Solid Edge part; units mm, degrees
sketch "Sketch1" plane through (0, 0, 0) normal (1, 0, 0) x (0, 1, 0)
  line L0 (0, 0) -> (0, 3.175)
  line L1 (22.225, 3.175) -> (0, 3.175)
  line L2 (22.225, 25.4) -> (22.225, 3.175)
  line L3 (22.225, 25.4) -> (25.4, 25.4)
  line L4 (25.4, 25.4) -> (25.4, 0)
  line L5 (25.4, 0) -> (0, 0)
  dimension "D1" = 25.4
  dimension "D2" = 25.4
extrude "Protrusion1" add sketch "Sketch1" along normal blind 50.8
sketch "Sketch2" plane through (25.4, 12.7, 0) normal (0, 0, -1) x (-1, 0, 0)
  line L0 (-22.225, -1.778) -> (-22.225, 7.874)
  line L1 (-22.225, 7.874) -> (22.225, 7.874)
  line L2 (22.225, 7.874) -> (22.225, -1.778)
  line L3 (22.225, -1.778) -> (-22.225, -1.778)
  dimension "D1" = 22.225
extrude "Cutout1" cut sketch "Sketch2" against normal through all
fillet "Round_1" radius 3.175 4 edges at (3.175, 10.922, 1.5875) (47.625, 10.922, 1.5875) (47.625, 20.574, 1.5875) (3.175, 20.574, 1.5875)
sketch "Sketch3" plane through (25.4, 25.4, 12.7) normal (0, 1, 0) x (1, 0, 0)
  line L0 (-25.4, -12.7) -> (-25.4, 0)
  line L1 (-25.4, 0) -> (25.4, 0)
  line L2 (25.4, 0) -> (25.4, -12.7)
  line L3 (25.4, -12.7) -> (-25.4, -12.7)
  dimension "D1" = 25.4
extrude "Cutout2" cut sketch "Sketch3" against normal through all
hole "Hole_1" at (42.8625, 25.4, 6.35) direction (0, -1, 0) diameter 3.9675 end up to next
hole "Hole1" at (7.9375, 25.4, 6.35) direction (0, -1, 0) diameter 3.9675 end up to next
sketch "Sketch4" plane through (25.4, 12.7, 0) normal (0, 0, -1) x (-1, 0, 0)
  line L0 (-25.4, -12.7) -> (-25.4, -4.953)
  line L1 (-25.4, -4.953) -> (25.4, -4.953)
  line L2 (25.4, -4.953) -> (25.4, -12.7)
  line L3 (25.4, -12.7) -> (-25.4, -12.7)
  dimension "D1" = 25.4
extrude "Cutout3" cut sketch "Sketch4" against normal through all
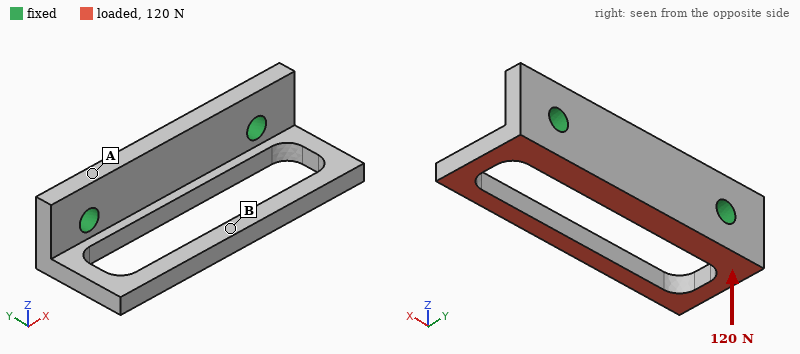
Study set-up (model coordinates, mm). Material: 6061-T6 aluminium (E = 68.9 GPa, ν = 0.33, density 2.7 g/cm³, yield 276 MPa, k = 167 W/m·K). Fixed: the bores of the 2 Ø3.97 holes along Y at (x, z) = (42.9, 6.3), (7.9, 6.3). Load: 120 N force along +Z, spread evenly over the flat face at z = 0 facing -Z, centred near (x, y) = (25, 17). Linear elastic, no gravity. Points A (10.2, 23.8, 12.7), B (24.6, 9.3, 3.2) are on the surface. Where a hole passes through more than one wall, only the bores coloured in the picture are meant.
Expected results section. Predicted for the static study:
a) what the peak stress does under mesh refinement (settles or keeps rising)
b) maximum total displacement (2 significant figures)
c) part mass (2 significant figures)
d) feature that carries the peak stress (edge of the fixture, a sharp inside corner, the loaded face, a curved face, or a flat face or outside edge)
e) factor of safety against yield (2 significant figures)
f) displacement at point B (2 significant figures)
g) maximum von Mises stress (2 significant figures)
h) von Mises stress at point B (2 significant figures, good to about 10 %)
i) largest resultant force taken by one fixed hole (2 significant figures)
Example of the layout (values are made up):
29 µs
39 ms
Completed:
settles
92 µm
8.0 g
the loaded face
5.9
85 µm
47 MPa
24 MPa
60 N
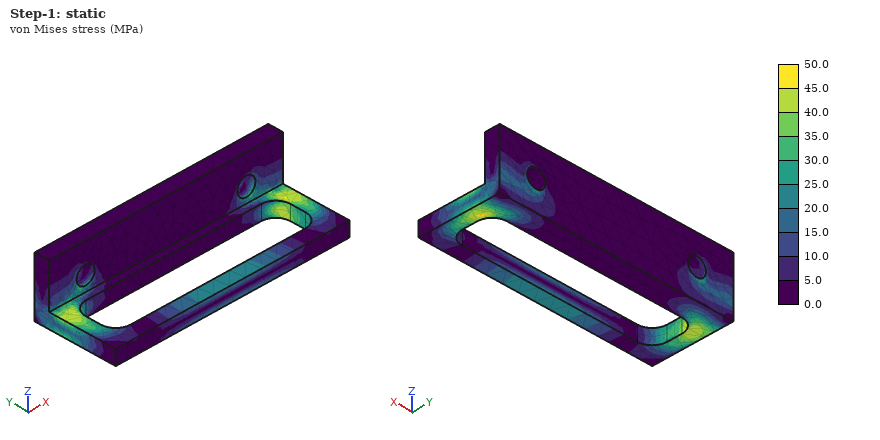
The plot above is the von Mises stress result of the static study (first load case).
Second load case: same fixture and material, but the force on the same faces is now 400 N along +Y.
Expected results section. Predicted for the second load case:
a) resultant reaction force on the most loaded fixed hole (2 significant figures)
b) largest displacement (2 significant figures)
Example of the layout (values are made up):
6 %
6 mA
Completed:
200 N
0.10 mm
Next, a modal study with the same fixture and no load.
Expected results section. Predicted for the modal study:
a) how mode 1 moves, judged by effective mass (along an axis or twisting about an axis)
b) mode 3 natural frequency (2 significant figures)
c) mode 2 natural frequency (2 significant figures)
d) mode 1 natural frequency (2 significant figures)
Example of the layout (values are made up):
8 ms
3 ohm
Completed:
along Z
6700 Hz
6500 Hz
3400 Hz
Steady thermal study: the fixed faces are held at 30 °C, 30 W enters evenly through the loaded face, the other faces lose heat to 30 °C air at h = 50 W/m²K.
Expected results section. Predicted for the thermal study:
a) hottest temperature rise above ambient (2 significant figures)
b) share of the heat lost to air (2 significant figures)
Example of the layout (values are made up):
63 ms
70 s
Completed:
70 K
7.0 %
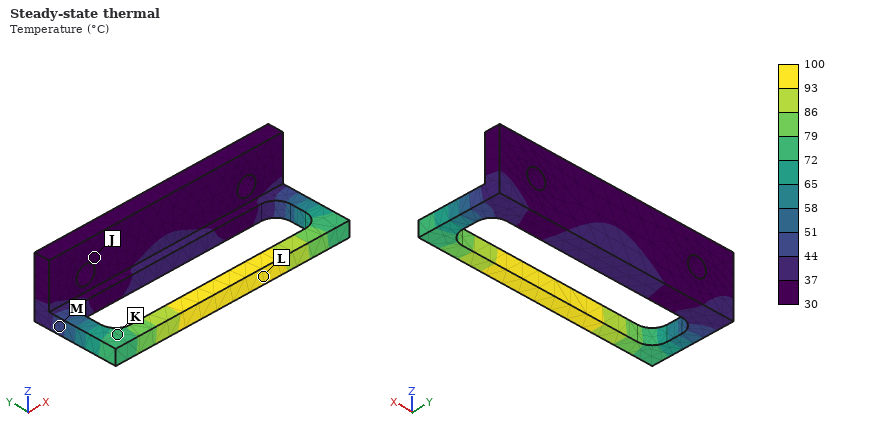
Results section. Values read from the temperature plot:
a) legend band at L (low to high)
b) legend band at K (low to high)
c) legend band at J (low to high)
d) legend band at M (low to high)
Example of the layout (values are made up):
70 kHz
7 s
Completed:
93 to 100 °C
72 to 79 °C
30 to 37 °C
44 to 51 °C
